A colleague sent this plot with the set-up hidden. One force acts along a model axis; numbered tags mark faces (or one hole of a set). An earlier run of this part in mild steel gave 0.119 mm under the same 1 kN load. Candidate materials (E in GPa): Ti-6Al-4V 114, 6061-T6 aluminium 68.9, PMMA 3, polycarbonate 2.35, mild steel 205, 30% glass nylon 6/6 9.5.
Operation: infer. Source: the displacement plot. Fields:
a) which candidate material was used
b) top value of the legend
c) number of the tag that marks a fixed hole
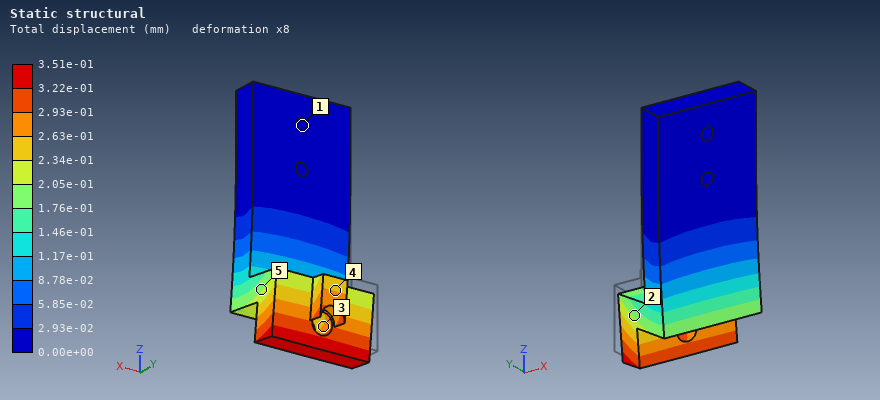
6061-T6 aluminium
3.51e-01 mm
1
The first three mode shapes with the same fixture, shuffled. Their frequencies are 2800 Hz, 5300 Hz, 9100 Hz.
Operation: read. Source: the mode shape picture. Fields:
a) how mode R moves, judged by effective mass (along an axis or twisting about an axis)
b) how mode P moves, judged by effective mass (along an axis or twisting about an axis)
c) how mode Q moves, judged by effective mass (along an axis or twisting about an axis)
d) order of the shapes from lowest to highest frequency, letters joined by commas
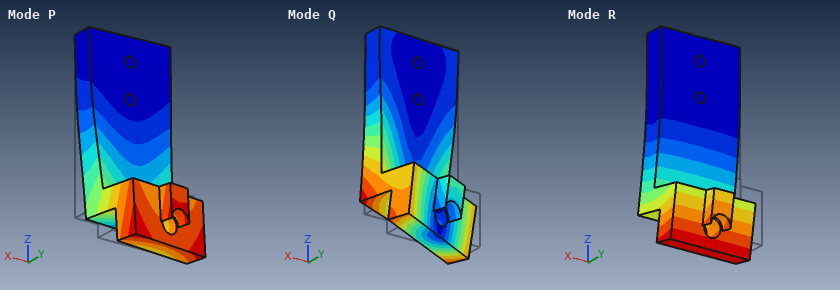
along Y
along X
along X
R, P, Q
